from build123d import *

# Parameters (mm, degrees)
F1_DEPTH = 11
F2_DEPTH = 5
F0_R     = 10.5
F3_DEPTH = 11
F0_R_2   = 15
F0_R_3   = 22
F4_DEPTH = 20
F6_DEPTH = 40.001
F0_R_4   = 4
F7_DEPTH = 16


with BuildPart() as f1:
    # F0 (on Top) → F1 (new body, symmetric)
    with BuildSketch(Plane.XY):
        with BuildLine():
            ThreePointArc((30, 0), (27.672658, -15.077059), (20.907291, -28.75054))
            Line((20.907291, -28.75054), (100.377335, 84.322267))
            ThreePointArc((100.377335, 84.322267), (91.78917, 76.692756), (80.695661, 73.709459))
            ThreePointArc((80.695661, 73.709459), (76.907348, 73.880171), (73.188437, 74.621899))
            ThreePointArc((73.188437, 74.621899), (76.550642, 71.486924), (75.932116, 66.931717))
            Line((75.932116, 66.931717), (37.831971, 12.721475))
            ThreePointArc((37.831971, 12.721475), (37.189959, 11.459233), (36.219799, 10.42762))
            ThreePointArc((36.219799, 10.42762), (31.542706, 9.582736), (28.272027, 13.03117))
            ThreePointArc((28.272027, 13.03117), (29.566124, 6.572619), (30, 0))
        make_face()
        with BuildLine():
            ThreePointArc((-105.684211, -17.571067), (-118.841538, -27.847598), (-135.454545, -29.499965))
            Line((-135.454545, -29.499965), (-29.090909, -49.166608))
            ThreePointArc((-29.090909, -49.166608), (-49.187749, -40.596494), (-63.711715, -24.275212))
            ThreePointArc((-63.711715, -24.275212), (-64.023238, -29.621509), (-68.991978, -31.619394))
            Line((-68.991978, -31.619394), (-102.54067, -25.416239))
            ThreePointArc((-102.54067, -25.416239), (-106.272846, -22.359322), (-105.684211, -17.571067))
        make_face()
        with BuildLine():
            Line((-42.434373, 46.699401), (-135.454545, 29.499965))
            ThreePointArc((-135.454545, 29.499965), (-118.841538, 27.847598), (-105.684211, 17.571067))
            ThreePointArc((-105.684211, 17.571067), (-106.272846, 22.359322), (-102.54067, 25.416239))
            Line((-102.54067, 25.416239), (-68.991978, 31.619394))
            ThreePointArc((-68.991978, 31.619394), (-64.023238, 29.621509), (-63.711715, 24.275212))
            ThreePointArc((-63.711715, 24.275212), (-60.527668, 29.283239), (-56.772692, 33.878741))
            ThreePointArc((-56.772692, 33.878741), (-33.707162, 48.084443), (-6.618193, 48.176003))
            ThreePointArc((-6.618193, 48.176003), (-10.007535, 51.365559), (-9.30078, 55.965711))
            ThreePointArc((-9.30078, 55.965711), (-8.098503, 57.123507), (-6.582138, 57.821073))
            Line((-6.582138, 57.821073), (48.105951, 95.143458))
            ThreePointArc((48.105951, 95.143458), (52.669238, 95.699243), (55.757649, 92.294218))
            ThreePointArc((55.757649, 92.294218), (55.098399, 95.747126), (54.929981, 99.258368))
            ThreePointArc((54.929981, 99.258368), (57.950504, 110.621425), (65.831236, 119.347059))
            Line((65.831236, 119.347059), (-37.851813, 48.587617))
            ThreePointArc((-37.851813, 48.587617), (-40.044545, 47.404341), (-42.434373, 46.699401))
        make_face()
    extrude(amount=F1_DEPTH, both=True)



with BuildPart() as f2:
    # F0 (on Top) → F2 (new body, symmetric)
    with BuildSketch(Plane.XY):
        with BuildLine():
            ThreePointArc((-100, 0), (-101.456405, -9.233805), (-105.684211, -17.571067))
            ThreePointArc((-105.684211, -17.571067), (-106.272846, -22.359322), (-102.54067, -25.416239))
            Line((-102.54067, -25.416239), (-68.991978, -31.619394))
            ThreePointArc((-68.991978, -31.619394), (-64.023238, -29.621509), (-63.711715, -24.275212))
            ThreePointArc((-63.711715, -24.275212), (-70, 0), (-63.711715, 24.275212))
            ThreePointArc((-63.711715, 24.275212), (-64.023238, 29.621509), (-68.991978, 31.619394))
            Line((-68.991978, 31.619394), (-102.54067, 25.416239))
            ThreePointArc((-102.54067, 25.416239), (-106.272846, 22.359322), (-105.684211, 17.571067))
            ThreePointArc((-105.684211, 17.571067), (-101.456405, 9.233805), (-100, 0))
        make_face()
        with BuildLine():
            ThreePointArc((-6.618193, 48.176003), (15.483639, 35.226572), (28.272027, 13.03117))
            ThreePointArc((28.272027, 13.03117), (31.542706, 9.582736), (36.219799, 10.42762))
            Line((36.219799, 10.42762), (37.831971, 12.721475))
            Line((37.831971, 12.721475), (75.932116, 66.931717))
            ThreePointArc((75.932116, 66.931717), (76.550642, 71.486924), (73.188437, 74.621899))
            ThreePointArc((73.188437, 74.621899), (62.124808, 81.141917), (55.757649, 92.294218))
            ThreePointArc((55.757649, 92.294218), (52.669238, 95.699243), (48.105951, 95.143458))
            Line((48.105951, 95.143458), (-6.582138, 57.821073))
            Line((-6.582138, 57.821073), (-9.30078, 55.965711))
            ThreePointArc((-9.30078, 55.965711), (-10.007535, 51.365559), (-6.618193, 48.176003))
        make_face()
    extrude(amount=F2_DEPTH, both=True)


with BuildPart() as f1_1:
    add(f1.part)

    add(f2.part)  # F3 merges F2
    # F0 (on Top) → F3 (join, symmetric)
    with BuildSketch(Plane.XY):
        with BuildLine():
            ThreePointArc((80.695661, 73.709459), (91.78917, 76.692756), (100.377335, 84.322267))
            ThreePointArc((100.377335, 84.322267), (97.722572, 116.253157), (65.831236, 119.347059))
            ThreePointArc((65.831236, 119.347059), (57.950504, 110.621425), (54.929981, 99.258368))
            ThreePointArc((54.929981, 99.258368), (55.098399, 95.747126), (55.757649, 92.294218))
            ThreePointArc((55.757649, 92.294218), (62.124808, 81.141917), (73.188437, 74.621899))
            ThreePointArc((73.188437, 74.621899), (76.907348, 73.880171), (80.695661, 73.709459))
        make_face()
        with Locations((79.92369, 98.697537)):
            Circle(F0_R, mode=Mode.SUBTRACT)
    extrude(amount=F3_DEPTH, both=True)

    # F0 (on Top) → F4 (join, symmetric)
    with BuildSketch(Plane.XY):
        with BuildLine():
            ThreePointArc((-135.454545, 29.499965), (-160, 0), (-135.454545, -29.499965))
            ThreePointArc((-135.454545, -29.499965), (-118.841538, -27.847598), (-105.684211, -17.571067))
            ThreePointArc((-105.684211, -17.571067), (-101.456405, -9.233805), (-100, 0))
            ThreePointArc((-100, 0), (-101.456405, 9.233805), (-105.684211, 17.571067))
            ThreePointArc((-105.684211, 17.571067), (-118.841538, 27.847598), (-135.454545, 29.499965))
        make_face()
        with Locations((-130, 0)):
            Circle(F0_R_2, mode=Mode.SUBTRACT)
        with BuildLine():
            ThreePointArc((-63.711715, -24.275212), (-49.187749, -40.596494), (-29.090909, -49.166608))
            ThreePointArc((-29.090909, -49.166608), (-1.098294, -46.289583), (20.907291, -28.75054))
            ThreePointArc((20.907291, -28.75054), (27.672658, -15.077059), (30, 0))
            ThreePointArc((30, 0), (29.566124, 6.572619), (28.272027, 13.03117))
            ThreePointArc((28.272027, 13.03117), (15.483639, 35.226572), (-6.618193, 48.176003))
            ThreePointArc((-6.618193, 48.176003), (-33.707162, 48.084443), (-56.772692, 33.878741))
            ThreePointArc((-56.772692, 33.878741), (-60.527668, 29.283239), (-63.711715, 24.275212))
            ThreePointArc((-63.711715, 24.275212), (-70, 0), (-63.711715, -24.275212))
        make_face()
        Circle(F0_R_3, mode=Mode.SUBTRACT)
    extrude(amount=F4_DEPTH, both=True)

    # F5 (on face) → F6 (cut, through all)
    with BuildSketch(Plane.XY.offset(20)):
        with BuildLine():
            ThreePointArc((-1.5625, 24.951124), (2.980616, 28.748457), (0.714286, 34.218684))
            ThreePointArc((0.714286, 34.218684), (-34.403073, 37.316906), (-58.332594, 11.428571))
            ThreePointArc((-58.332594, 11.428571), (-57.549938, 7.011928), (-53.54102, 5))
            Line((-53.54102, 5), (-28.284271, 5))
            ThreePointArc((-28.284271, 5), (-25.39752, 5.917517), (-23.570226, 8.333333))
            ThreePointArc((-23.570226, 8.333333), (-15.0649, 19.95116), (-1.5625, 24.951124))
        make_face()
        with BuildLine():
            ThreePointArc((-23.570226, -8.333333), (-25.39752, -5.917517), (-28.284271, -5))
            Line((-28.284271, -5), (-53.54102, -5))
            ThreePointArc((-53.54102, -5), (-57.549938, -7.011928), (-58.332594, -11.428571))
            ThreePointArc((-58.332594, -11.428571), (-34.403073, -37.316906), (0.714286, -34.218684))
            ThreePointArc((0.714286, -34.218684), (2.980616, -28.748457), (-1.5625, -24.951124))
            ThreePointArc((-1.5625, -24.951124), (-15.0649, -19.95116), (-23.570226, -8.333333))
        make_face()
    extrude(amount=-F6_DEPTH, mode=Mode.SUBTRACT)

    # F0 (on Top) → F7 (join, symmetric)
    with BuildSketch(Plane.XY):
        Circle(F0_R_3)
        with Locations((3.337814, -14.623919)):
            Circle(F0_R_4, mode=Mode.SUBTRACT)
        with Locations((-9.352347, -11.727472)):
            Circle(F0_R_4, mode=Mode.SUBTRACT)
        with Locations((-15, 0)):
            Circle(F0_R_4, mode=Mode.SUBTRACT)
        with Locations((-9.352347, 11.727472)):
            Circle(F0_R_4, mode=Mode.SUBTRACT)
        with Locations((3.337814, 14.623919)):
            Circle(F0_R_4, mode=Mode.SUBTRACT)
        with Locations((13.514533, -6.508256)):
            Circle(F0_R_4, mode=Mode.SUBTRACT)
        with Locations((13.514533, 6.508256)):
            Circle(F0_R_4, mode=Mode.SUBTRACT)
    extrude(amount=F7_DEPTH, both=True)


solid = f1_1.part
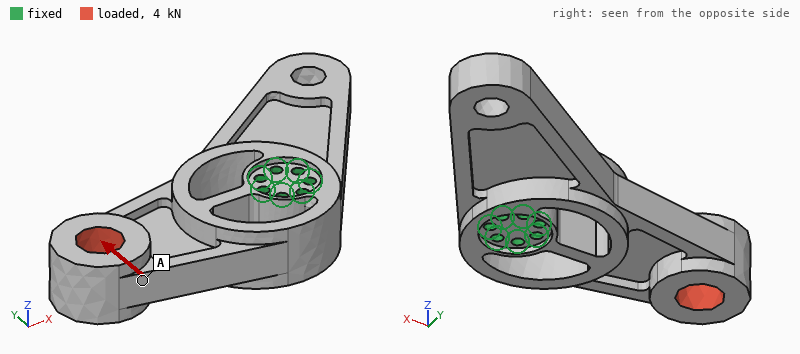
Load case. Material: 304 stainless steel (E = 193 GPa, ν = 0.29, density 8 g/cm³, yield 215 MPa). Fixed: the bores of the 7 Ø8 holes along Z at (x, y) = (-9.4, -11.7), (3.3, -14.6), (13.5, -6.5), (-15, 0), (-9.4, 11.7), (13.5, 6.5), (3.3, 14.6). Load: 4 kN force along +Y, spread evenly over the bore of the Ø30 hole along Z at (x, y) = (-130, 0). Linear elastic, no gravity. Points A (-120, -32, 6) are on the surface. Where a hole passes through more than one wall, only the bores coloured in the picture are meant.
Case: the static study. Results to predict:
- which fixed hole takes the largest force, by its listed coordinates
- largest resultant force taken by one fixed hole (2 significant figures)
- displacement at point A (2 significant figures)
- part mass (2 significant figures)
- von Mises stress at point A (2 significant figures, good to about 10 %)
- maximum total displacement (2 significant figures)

(3.3, 14.6)
8.2 kN
48 µm
3.5 kg
5.5 MPa
62 µm
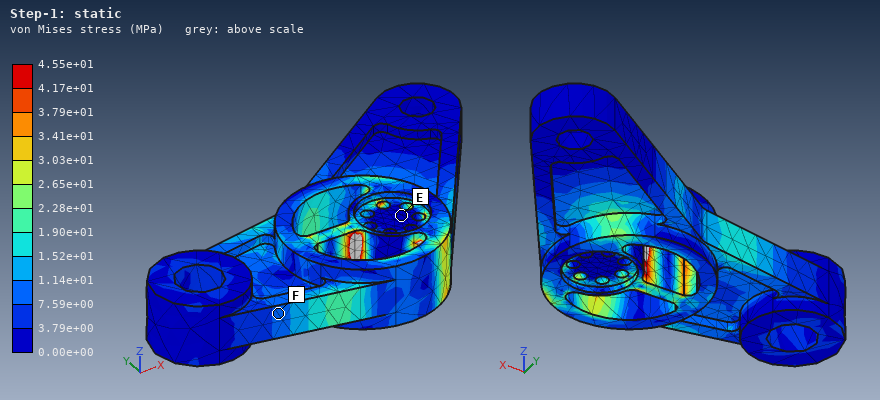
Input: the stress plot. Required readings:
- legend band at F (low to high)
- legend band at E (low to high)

7.59e+00 to 1.14e+01 MPa
0.00e+00 to 3.79e+00 MPa
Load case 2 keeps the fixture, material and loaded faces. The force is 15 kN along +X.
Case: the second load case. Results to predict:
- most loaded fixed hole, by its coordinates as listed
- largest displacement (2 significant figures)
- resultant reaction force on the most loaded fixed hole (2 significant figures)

(-15, 0)
14 µm
6.9 kN
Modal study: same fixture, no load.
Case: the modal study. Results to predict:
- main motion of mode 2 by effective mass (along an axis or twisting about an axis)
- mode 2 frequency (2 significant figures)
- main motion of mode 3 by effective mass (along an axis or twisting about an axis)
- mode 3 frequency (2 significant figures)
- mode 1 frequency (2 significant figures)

along Z
870 Hz
along Y
1300 Hz
760 Hz
